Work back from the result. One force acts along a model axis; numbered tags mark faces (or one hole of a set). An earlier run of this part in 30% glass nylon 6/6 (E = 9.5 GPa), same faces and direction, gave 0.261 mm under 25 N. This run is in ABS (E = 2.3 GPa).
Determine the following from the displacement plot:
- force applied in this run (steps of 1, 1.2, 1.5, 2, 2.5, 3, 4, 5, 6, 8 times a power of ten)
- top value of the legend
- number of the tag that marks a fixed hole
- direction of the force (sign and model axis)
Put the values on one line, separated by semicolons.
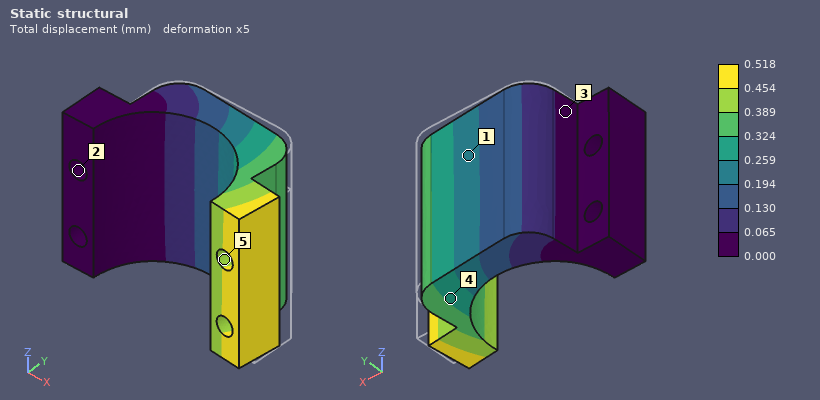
12 N; 0.518 mm; 2; -Y
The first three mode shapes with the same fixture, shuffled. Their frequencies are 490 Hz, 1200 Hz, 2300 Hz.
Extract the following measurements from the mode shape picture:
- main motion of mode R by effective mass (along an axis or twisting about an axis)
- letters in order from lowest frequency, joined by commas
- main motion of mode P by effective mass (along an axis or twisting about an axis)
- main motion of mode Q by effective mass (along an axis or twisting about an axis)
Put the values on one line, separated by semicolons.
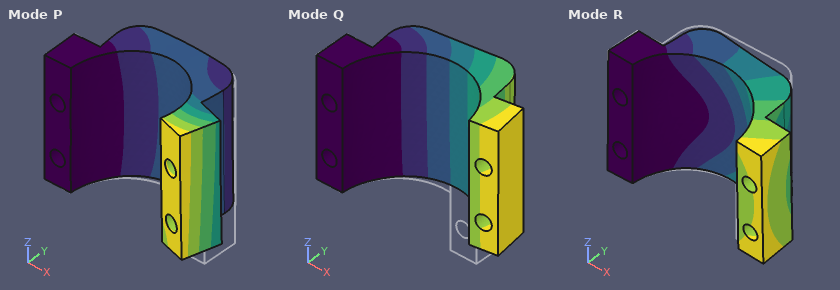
along Z; Q, R, P; along X; along Y
